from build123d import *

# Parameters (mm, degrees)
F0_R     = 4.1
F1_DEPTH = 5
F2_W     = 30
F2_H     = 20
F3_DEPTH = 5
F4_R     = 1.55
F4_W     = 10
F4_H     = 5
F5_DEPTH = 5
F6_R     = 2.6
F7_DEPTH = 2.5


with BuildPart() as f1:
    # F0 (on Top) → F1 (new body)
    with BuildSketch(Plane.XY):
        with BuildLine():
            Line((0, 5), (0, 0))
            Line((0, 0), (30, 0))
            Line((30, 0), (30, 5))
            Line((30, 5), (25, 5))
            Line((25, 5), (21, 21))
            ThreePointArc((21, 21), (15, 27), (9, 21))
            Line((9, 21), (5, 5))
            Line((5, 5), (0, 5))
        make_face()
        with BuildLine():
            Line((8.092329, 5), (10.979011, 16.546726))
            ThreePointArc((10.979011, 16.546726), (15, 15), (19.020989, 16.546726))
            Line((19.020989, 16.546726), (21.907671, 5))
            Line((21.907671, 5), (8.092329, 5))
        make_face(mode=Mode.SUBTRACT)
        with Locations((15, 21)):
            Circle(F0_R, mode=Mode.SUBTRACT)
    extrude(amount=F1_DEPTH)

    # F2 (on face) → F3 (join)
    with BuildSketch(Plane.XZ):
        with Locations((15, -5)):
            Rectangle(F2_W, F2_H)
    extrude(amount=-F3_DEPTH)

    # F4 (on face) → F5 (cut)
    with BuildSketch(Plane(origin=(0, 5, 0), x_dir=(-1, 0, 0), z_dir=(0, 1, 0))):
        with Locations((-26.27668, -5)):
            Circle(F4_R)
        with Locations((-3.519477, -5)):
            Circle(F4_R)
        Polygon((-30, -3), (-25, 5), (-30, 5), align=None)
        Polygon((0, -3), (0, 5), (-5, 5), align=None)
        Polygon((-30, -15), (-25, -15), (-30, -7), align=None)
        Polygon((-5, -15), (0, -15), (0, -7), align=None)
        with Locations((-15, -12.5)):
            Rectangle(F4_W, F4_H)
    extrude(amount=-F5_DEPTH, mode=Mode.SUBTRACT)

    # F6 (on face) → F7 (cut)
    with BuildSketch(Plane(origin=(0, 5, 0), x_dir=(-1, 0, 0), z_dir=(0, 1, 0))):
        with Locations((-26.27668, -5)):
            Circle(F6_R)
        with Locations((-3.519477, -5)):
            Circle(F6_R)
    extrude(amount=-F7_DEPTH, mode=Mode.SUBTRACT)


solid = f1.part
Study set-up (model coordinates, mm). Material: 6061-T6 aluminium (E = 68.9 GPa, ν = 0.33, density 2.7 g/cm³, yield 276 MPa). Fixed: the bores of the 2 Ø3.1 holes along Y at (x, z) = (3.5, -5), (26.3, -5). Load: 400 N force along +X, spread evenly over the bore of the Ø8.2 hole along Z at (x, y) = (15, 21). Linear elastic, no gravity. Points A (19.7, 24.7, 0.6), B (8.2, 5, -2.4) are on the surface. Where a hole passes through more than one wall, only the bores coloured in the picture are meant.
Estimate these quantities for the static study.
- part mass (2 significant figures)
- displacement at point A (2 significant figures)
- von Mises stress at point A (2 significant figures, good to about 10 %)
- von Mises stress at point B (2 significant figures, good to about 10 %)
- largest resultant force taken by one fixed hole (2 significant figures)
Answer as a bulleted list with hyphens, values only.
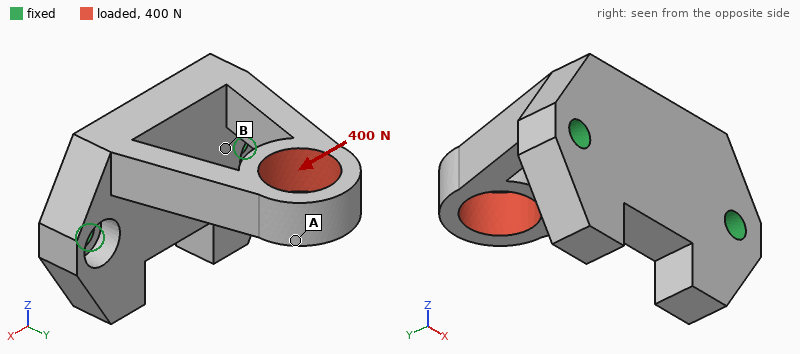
- 7.9 g
- 0.10 mm
- 68 MPa
- 31 MPa
- 420 N
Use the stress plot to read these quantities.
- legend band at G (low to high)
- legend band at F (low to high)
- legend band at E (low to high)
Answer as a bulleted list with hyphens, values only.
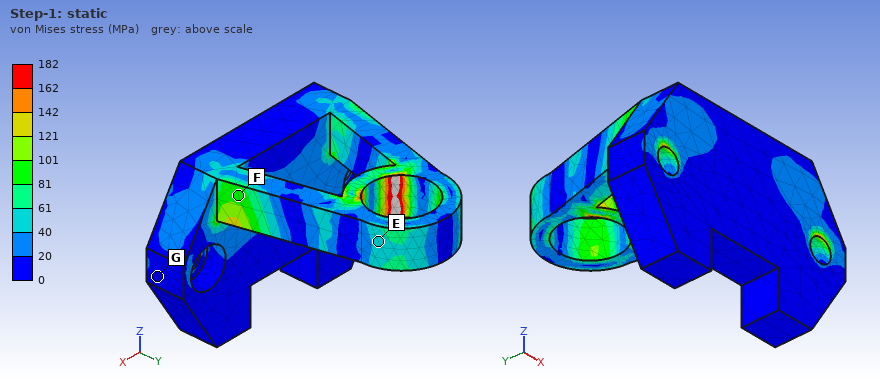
- 0 to 20 MPa
- 81 to 101 MPa
- 40 to 61 MPa
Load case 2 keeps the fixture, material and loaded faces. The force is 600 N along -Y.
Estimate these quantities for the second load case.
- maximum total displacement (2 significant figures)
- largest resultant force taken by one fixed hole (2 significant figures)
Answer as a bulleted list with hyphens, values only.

- 86 µm
- 320 N
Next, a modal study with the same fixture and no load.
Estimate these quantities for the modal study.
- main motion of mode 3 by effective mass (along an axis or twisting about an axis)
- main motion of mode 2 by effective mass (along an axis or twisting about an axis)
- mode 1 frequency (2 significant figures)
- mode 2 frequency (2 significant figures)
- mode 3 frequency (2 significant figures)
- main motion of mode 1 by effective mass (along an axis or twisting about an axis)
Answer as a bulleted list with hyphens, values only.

- along Y
- along X
- 5200 Hz
- 9900 Hz
- 15 kHz
- along Z
